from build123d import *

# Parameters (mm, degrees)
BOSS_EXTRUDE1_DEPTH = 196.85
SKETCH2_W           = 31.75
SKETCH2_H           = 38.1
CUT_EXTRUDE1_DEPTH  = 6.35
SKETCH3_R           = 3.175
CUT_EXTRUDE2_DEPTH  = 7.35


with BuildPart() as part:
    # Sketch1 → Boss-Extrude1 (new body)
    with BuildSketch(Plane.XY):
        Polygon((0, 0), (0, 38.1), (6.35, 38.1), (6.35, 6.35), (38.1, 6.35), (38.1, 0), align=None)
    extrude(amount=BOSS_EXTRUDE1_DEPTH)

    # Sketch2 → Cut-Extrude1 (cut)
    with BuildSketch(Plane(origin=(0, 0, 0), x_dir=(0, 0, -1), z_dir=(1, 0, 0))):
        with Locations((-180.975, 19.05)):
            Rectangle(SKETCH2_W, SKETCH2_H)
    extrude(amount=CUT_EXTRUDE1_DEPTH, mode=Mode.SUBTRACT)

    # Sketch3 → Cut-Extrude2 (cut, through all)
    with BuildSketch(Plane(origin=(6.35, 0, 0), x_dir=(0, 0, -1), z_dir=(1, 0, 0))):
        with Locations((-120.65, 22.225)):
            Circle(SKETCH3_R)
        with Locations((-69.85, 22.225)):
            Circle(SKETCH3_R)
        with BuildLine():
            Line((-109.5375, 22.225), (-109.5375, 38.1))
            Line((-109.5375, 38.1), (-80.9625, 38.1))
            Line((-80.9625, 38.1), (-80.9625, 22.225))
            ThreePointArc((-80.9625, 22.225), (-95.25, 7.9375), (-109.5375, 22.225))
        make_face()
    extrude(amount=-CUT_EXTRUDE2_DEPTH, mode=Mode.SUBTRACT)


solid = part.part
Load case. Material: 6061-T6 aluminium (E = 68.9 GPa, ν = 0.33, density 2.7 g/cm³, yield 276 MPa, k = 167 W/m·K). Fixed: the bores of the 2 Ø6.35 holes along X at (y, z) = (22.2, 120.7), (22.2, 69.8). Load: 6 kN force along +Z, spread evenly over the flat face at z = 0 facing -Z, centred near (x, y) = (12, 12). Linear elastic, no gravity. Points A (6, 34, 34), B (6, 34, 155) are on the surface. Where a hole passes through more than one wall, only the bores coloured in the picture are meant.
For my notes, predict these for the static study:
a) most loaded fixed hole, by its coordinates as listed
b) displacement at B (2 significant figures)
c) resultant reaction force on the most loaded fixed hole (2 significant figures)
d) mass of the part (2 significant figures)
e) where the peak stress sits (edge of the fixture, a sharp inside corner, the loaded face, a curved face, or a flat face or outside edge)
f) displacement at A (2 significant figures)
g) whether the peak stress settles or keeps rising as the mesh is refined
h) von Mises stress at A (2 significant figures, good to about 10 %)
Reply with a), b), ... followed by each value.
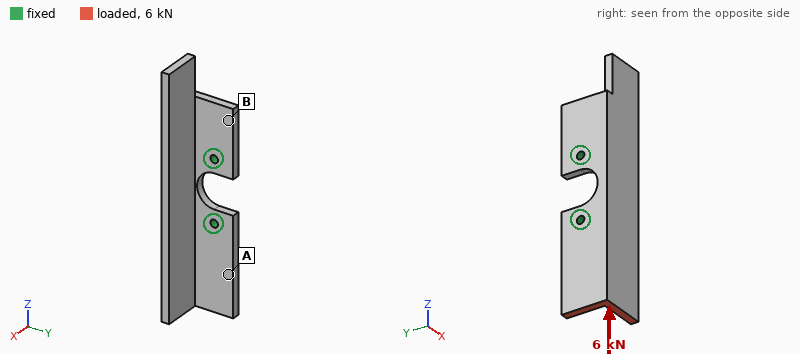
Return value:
a) (22.2, 69.8)
b) 0.019 mm
c) 4.5 kN
d) 200 g
e) edge of the fixture
f) 0.023 mm
g) keeps rising
h) 16 MPa
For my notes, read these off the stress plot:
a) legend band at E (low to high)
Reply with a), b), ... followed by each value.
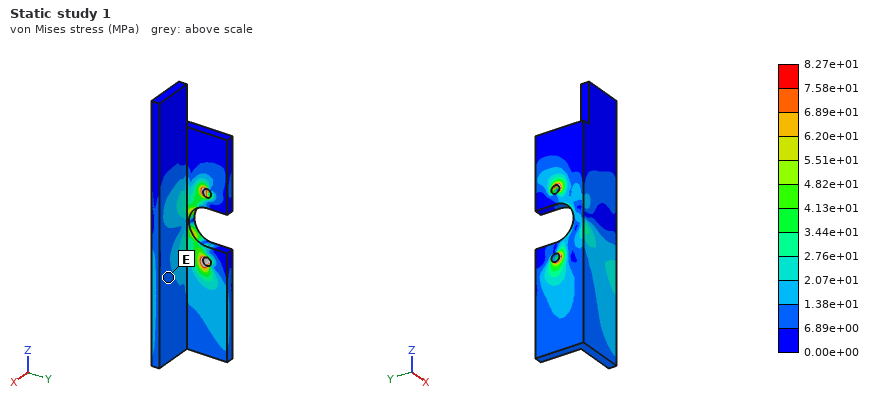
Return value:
a) 6.89e+00 to 1.38e+01 MPa
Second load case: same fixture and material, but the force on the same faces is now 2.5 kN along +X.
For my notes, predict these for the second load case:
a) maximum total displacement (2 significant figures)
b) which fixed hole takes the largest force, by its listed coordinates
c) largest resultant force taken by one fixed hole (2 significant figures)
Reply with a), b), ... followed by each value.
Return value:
a) 0.69 mm
b) (22.2, 69.8)
c) 4.9 kN
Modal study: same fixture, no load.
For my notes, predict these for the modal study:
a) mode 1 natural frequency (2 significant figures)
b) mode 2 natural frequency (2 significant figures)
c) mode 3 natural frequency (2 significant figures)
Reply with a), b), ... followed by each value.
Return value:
a) 1300 Hz
b) 1500 Hz
c) 1900 Hz
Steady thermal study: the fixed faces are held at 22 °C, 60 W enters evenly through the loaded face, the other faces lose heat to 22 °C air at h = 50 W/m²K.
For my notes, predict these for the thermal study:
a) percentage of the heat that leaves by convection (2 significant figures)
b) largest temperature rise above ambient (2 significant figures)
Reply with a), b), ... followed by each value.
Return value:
a) 32 %
b) 56 K
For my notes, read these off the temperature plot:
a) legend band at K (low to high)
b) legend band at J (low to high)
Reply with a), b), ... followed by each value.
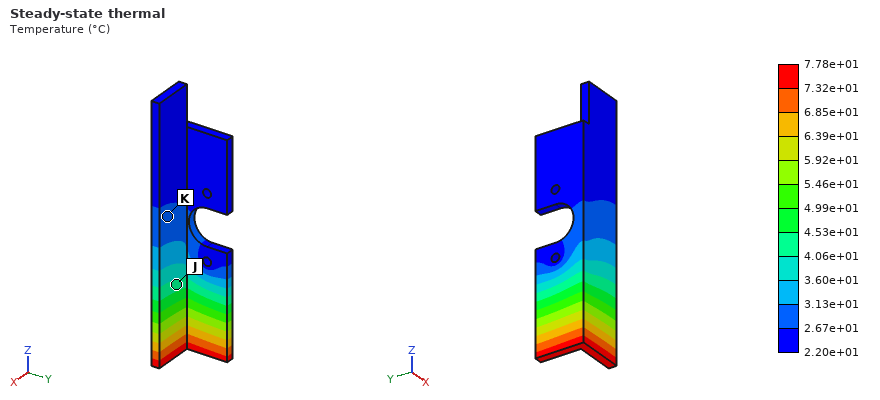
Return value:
a) 2.67e+01 to 3.13e+01 °C
b) 4.06e+01 to 4.53e+01 °C
